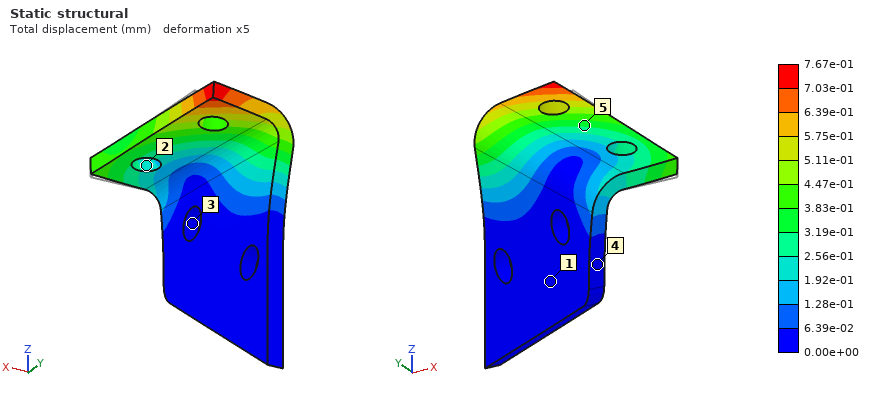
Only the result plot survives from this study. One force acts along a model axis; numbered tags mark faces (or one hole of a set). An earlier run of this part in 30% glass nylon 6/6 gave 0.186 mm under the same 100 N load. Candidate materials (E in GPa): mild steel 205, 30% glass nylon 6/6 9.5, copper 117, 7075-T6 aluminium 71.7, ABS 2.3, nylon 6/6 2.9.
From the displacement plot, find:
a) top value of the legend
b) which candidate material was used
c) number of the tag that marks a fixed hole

7.67e-01 mm
ABS
3
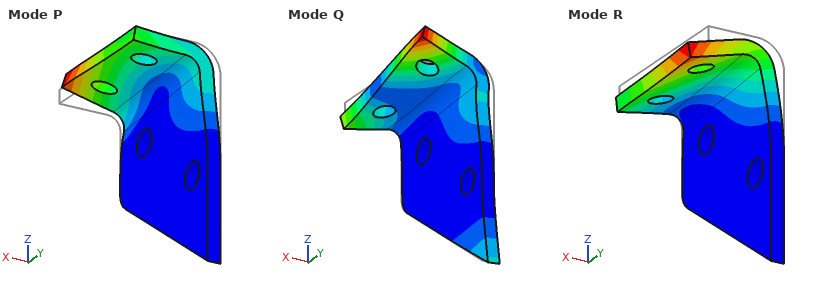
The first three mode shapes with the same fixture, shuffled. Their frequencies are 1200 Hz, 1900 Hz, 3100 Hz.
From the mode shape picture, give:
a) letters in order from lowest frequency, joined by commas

R, P, Q
